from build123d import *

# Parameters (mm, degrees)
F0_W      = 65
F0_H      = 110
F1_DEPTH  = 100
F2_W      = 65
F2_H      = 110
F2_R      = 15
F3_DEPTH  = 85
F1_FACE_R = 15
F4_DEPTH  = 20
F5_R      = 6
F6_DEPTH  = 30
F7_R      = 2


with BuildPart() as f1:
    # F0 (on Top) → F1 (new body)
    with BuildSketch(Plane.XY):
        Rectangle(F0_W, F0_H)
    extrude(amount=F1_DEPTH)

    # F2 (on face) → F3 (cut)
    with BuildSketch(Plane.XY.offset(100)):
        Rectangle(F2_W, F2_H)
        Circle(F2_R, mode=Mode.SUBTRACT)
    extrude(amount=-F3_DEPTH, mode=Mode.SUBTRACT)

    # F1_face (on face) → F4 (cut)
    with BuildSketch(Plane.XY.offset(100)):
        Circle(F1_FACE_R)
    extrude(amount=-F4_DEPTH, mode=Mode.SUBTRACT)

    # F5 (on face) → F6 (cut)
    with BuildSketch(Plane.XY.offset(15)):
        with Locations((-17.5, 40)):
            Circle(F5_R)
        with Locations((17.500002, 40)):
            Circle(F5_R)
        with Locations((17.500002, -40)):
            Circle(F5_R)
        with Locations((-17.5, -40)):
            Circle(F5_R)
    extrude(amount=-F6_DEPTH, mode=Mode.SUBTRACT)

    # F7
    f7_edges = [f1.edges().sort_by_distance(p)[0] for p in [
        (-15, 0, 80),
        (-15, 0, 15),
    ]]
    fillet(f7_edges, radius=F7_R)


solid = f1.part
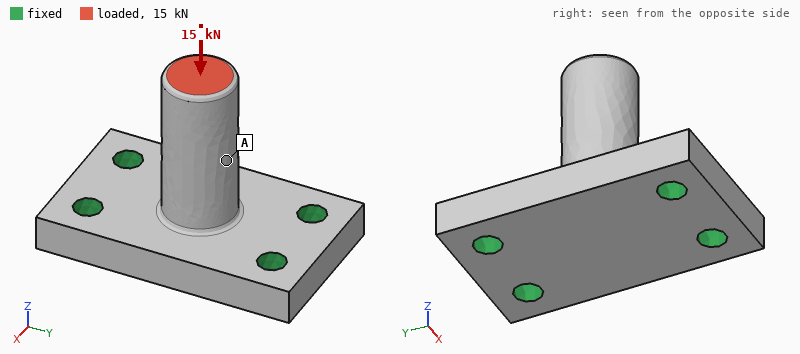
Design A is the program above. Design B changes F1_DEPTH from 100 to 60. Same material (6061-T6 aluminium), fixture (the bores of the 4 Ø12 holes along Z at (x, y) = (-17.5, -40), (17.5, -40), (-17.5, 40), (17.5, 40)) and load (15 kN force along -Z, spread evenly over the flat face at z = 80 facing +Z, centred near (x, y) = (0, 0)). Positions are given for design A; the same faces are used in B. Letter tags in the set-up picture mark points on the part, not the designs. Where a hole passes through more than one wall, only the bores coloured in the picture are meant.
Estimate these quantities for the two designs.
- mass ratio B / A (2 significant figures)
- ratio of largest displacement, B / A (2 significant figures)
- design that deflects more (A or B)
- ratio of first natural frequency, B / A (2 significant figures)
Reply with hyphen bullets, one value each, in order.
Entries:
- 0.90
- 0.87
- A
- 1.7
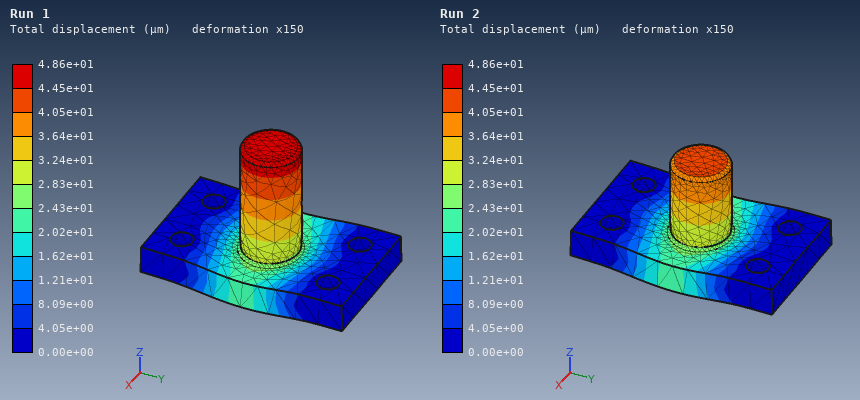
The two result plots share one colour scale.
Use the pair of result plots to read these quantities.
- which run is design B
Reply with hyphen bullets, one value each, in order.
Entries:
- Run 2
